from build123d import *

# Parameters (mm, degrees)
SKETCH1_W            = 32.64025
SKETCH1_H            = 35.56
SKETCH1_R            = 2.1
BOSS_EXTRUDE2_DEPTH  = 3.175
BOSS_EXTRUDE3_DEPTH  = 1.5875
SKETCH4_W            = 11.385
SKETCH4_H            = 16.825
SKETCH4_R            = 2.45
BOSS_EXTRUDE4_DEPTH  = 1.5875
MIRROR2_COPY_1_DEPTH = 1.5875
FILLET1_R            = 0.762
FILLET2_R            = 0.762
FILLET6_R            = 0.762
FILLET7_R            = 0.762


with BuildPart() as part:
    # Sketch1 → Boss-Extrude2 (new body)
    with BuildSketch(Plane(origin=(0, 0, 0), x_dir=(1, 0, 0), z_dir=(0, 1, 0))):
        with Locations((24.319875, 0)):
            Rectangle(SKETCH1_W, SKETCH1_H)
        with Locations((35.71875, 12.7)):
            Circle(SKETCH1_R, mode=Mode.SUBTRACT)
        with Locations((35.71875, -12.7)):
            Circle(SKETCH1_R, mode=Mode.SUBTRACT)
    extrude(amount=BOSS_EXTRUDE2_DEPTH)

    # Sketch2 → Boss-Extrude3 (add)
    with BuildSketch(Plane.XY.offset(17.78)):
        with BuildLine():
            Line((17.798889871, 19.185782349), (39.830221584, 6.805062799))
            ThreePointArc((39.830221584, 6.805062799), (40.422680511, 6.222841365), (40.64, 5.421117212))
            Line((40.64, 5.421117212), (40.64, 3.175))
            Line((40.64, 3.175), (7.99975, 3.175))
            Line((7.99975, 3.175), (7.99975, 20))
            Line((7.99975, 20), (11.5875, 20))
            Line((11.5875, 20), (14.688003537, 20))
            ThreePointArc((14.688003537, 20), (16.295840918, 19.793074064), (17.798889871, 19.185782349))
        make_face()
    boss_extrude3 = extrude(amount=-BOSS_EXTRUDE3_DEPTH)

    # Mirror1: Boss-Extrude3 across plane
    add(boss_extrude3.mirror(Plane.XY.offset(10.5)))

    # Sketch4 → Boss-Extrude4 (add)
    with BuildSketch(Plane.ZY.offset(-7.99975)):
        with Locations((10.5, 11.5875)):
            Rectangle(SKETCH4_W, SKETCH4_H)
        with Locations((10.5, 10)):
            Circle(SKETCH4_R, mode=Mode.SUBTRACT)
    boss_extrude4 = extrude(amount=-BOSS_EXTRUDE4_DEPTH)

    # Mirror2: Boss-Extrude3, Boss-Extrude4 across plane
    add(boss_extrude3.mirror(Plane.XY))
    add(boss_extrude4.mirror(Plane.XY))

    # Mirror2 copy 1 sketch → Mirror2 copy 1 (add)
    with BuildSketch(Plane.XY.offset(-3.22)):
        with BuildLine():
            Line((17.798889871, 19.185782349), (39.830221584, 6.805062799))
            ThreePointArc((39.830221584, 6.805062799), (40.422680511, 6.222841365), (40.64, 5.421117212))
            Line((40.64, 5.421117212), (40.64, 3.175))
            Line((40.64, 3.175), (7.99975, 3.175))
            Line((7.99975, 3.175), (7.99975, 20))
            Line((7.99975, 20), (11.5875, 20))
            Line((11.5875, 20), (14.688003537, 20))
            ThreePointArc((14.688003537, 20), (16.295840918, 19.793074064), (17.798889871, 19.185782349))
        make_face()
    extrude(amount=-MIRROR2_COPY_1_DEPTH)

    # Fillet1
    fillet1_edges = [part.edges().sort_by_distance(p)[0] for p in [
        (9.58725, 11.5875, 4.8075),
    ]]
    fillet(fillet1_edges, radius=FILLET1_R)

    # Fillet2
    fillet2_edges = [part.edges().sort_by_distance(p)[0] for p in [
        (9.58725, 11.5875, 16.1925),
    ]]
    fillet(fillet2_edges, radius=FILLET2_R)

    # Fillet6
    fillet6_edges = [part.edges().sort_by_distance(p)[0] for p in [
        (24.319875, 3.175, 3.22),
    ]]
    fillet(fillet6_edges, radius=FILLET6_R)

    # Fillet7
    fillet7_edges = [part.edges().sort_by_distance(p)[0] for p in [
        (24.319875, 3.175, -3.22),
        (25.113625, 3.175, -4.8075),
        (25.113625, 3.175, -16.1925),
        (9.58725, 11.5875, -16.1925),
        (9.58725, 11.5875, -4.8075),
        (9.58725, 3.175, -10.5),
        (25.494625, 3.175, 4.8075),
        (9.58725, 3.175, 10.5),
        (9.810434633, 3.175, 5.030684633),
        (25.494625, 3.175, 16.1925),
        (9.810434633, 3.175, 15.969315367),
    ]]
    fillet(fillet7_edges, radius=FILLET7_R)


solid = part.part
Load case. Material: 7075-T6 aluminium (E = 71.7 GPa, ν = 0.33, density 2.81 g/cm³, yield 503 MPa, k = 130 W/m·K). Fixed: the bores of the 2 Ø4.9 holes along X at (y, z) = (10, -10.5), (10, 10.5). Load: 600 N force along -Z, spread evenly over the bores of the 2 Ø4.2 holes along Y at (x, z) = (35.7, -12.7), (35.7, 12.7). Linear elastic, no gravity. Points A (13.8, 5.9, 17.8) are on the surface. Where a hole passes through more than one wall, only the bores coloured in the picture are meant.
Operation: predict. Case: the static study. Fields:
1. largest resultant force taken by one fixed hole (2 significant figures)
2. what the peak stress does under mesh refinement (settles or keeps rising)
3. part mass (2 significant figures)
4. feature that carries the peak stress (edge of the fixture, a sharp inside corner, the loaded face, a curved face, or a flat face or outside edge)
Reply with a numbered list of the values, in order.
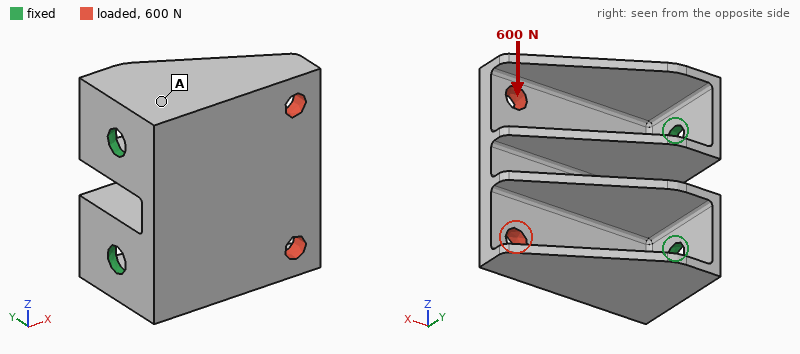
1. 780 N
2. keeps rising
3. 19 g
4. edge of the fixture
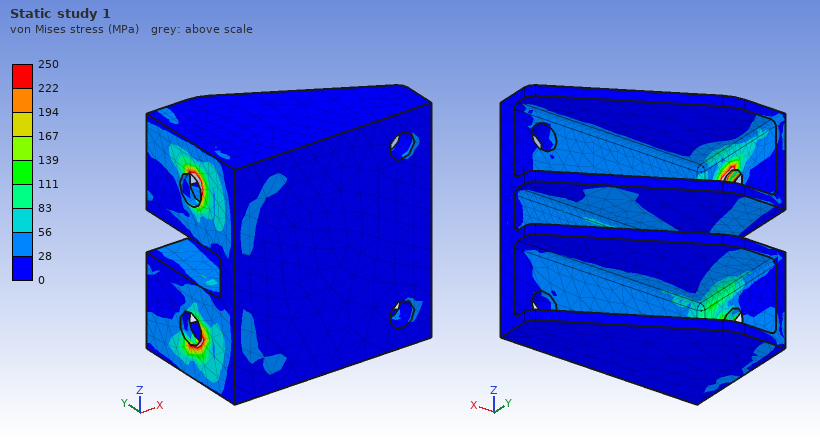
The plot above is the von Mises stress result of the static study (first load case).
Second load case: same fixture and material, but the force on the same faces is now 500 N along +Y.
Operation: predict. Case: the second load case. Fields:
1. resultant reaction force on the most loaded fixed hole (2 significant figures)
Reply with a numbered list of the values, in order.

1. 250 N
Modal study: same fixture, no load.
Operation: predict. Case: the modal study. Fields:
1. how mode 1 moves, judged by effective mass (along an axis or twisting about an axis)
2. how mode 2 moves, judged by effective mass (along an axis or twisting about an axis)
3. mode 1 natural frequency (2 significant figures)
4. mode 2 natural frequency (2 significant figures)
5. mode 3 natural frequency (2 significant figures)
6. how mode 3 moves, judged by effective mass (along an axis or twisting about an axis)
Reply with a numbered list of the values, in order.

1. along Y
2. along Z
3. 2200 Hz
4. 3500 Hz
5. 7200 Hz
6. along Z
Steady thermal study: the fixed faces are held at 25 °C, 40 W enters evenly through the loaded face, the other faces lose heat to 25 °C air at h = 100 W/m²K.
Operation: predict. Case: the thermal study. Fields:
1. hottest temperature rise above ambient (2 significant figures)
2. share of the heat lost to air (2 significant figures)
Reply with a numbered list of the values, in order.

1. 60 K
2. 39 %
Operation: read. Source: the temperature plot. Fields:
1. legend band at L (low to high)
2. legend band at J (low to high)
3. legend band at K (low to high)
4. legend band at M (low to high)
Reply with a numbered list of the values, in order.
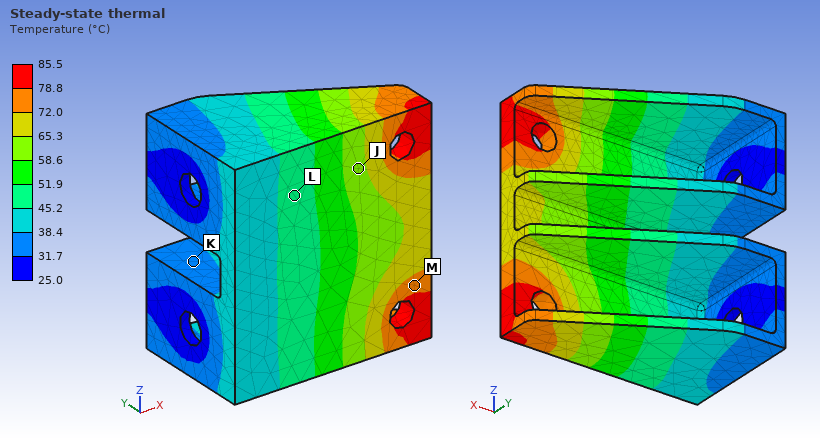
1. 45.2 to 51.9 °C
2. 58.6 to 65.3 °C
3. 31.7 to 38.4 °C
4. 72.0 to 78.8 °C
